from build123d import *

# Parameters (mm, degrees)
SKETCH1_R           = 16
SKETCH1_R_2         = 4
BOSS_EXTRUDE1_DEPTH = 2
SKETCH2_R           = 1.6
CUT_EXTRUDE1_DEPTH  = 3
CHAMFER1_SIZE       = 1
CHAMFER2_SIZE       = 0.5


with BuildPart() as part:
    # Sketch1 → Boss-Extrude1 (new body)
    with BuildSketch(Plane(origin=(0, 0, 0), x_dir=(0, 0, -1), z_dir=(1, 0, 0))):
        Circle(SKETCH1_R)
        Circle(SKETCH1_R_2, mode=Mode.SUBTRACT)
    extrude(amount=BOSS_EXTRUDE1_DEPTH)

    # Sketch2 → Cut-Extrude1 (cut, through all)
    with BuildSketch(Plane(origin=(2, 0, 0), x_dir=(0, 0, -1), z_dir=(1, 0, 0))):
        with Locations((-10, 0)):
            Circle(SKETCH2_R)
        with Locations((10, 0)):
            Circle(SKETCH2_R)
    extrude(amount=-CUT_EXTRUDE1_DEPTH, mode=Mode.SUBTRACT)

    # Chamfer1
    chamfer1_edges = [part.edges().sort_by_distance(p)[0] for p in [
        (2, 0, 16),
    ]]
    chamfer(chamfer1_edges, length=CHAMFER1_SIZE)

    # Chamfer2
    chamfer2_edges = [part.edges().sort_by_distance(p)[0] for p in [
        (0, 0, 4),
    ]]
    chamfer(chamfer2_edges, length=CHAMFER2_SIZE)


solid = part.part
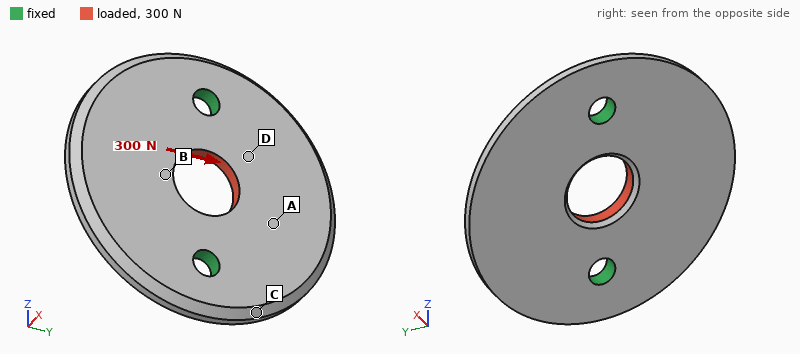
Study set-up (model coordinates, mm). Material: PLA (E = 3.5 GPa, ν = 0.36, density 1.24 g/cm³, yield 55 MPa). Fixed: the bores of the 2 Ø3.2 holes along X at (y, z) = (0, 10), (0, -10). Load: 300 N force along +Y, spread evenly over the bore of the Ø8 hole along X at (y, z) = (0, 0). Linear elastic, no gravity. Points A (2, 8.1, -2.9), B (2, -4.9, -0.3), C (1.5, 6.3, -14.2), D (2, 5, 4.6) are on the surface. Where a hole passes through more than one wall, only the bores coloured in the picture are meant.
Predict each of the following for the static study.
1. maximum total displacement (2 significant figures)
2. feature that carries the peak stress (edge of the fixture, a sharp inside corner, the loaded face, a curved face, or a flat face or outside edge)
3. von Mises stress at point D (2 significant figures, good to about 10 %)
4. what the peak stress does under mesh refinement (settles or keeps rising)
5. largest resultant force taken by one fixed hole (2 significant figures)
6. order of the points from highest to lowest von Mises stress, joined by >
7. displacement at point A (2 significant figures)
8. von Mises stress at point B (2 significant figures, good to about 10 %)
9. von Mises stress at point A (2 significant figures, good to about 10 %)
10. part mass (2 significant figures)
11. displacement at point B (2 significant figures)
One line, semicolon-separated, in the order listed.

47 µm; edge of the fixture; 6.5 MPa; keeps rising; 150 N; B > D > A > C; 30 µm; 8.5 MPa; 4.3 MPa; 1.8 g; 31 µm
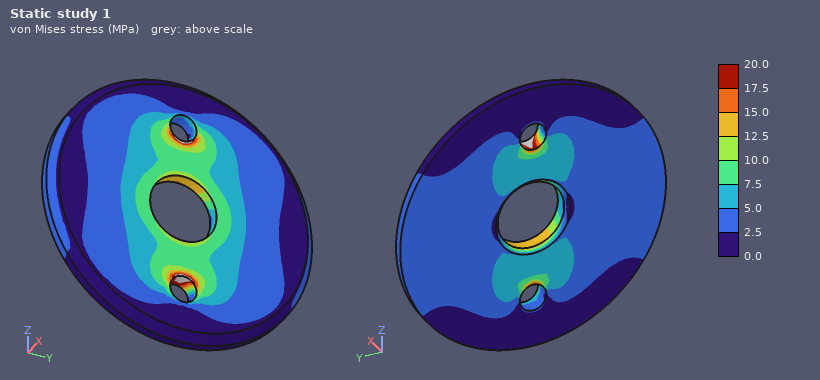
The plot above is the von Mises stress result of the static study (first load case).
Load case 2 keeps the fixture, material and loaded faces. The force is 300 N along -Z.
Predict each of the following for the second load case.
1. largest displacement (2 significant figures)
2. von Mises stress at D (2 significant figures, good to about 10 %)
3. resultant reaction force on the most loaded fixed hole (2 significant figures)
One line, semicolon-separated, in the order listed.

22 µm; 4.2 MPa; 150 N
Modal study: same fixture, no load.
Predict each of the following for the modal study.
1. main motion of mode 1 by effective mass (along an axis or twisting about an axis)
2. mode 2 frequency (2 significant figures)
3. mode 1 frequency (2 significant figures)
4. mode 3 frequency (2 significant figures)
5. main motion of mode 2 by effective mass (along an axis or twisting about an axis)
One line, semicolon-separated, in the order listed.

twisting about Z; 2700 Hz; 2500 Hz; 5900 Hz; along X
